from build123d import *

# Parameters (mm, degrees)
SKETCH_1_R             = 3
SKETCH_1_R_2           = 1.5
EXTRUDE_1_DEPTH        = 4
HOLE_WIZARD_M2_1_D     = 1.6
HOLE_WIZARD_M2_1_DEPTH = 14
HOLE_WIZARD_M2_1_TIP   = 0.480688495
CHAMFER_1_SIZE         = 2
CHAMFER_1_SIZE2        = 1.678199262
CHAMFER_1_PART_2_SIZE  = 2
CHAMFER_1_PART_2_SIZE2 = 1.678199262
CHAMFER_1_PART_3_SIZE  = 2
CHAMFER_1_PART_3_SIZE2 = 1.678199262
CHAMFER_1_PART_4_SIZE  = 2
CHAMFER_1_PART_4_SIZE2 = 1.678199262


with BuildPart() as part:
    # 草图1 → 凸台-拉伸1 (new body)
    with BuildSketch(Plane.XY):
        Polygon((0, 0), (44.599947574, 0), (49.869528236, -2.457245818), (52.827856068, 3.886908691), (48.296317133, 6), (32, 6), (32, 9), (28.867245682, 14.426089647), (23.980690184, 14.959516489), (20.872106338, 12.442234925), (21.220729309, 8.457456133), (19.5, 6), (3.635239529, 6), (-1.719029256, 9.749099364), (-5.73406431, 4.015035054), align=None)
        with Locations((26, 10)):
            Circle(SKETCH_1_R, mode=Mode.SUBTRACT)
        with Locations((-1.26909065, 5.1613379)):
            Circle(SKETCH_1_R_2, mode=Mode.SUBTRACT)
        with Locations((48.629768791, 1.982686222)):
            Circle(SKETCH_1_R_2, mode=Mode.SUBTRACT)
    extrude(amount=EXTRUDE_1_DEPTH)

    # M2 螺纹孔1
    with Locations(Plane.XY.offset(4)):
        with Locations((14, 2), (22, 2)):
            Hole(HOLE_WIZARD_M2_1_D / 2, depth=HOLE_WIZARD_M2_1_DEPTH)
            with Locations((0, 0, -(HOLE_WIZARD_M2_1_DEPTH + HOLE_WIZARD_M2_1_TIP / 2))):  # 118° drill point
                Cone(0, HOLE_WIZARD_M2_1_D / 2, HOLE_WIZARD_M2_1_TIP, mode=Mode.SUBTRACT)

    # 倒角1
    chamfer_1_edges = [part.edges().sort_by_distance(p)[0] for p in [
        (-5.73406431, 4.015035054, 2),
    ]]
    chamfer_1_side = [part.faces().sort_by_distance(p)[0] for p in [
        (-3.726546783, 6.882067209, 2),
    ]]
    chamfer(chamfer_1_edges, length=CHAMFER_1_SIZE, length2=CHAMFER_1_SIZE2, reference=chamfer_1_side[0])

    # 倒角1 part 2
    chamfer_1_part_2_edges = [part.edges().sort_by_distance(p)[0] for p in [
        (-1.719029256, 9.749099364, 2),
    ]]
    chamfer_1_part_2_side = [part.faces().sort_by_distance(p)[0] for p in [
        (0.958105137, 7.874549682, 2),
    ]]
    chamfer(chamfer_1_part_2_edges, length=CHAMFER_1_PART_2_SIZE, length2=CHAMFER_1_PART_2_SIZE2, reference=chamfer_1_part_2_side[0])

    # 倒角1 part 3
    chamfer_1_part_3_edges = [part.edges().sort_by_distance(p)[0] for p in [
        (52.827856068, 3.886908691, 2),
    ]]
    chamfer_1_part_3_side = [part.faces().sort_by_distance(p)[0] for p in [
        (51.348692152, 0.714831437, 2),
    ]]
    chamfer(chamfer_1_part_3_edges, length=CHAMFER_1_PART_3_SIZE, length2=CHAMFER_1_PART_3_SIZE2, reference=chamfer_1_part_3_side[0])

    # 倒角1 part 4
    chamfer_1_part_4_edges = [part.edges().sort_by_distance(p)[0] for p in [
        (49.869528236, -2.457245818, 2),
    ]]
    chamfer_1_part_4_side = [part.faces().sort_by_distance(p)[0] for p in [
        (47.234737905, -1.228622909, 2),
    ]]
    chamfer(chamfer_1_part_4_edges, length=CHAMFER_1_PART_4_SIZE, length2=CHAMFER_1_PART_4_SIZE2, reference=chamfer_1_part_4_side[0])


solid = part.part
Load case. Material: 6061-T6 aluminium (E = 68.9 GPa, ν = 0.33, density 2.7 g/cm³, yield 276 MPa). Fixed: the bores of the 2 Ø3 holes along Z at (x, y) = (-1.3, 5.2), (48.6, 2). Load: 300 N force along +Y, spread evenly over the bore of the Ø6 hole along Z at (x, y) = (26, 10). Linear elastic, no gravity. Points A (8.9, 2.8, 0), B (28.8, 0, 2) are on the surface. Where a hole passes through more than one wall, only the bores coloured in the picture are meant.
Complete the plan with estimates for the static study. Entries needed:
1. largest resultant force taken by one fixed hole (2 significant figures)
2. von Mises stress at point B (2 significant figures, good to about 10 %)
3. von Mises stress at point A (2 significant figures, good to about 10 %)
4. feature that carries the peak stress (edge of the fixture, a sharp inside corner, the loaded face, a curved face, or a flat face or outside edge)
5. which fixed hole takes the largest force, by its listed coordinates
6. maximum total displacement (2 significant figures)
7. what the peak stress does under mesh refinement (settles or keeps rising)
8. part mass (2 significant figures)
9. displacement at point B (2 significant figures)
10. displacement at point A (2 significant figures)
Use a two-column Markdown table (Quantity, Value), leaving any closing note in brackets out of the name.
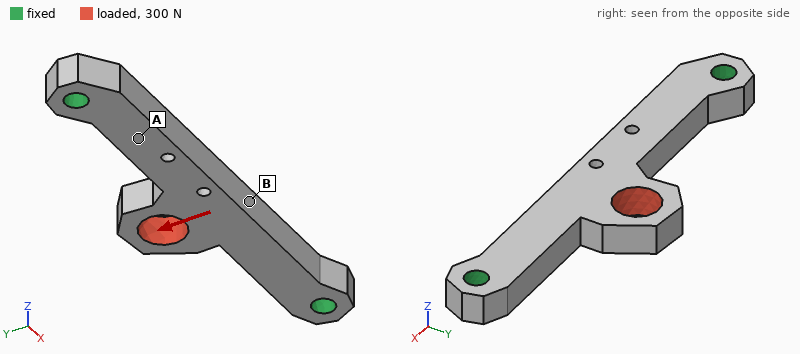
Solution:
| Quantity | Value |
|---|---|
| largest resultant force taken by one fixed hole | 170 N |
| von Mises stress at point B | 38 MPa |
| von Mises stress at point A | 15 MPa |
| feature that carries the peak stress | edge of the fixture |
| which fixed hole takes the largest force, by its listed coordinates | (48.6, 2) |
| maximum total displacement | 36 µm |
| what the peak stress does under mesh refinement | keeps rising |
| part mass | 4.2 g |
| displacement at point B | 32 µm |
| displacement at point A | 14 µm |
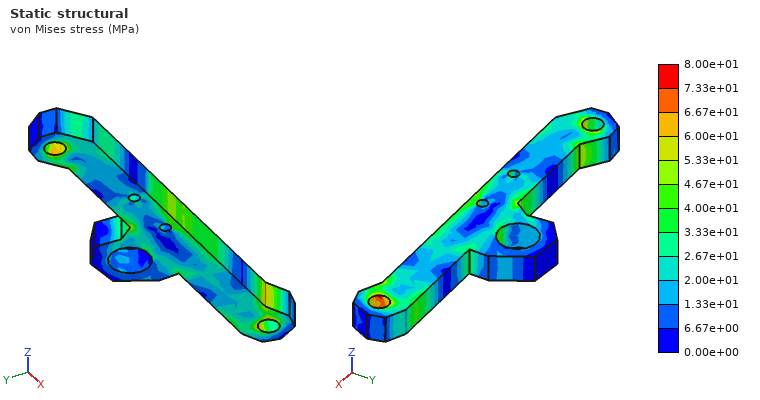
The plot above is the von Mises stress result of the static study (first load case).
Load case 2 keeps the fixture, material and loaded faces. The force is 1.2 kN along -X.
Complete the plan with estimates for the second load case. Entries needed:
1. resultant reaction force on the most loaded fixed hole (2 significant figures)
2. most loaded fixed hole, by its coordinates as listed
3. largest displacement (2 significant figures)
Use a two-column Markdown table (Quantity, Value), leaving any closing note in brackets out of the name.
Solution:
| Quantity | Value |
|---|---|
| resultant reaction force on the most loaded fixed hole | 790 N |
| most loaded fixed hole, by its coordinates as listed | (48.6, 2) |
| largest displacement | 74 µm |
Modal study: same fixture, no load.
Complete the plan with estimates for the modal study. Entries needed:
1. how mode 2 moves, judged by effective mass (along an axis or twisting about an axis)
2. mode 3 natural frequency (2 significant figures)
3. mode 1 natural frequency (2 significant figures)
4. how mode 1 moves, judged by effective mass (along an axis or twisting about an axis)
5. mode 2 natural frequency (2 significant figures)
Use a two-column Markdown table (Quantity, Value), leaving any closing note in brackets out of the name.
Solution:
| Quantity | Value |
|---|---|
| how mode 2 moves, judged by effective mass | along Y |
| mode 3 natural frequency | 13 kHz |
| mode 1 natural frequency | 6800 Hz |
| how mode 1 moves, judged by effective mass | along Z |
| mode 2 natural frequency | 10 kHz |
